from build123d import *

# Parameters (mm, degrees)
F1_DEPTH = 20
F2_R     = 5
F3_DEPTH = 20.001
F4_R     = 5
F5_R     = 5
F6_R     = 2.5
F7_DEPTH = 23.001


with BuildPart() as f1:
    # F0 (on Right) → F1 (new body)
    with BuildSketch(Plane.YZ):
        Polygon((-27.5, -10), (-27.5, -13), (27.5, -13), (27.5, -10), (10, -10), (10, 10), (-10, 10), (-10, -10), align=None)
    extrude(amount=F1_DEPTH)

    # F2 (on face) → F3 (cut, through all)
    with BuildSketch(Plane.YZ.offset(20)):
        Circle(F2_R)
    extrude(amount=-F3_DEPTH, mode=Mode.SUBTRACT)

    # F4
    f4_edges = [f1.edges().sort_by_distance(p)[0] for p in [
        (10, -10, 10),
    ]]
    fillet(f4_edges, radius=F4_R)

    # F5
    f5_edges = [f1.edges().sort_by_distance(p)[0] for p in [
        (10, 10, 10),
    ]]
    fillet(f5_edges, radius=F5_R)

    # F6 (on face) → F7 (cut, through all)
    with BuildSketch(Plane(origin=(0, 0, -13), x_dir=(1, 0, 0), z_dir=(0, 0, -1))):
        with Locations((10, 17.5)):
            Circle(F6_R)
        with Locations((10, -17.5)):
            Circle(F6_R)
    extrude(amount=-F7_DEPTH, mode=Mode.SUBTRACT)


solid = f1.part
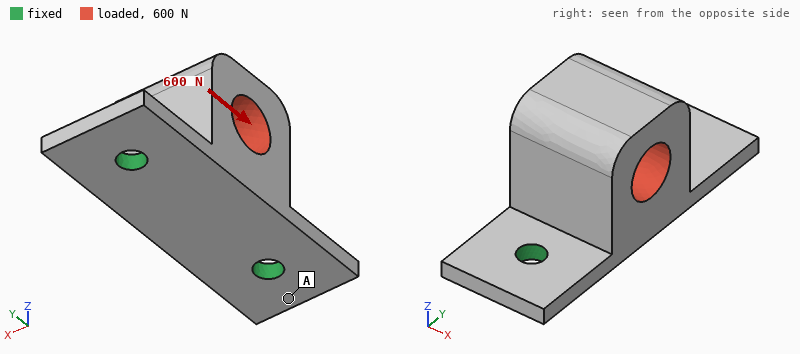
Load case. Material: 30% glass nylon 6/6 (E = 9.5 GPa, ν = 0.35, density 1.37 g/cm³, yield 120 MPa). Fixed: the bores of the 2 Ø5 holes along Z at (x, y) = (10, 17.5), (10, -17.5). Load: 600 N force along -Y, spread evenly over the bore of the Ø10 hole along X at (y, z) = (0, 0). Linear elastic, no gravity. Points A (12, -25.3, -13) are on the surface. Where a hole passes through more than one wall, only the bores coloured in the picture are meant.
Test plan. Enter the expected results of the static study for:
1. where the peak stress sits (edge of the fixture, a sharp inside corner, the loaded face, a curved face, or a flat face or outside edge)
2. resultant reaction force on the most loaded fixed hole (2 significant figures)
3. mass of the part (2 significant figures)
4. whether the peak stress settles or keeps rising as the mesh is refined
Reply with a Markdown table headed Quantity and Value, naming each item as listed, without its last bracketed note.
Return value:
| Quantity | Value |
|---|---|
| where the peak stress sits | edge of the fixture |
| resultant reaction force on the most loaded fixed hole | 400 N |
| mass of the part | 13 g |
| whether the peak stress settles or keeps rising as the mesh is refined | keeps rising |
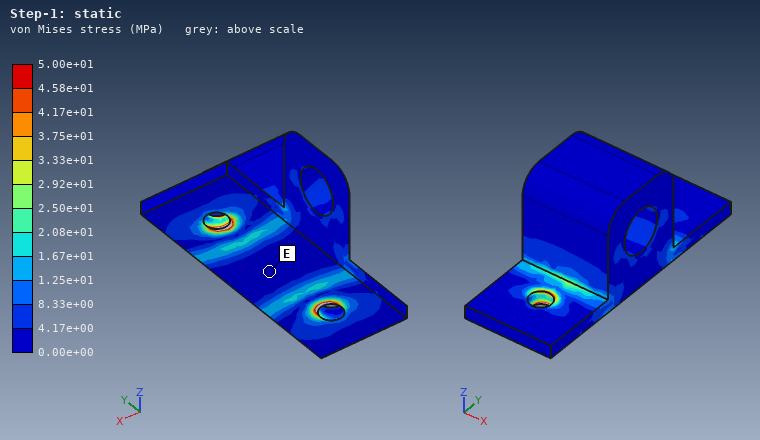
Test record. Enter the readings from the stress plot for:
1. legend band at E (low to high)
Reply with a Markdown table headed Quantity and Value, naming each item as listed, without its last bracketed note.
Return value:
| Quantity | Value |
|---|---|
| legend band at E | 0.00e+00 to 4.17e+00 MPa |
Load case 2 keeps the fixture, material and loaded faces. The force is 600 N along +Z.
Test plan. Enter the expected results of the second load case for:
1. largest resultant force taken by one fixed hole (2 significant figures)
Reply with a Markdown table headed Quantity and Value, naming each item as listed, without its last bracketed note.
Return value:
| Quantity | Value |
|---|---|
| largest resultant force taken by one fixed hole | 330 N |
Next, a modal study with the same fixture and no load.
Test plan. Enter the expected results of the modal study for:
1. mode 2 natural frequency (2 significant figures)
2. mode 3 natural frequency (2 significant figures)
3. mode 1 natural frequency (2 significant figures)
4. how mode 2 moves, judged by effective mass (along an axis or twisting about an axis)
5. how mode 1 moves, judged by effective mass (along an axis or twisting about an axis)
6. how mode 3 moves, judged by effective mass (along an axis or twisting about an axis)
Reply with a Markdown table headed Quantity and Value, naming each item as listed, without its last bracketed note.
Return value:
| Quantity | Value |
|---|---|
| mode 2 natural frequency | 4900 Hz |
| mode 3 natural frequency | 5200 Hz |
| mode 1 natural frequency | 1900 Hz |
| how mode 2 moves, judged by effective mass | along Y |
| how mode 1 moves, judged by effective mass | along X |
| how mode 3 moves, judged by effective mass | along Z |
